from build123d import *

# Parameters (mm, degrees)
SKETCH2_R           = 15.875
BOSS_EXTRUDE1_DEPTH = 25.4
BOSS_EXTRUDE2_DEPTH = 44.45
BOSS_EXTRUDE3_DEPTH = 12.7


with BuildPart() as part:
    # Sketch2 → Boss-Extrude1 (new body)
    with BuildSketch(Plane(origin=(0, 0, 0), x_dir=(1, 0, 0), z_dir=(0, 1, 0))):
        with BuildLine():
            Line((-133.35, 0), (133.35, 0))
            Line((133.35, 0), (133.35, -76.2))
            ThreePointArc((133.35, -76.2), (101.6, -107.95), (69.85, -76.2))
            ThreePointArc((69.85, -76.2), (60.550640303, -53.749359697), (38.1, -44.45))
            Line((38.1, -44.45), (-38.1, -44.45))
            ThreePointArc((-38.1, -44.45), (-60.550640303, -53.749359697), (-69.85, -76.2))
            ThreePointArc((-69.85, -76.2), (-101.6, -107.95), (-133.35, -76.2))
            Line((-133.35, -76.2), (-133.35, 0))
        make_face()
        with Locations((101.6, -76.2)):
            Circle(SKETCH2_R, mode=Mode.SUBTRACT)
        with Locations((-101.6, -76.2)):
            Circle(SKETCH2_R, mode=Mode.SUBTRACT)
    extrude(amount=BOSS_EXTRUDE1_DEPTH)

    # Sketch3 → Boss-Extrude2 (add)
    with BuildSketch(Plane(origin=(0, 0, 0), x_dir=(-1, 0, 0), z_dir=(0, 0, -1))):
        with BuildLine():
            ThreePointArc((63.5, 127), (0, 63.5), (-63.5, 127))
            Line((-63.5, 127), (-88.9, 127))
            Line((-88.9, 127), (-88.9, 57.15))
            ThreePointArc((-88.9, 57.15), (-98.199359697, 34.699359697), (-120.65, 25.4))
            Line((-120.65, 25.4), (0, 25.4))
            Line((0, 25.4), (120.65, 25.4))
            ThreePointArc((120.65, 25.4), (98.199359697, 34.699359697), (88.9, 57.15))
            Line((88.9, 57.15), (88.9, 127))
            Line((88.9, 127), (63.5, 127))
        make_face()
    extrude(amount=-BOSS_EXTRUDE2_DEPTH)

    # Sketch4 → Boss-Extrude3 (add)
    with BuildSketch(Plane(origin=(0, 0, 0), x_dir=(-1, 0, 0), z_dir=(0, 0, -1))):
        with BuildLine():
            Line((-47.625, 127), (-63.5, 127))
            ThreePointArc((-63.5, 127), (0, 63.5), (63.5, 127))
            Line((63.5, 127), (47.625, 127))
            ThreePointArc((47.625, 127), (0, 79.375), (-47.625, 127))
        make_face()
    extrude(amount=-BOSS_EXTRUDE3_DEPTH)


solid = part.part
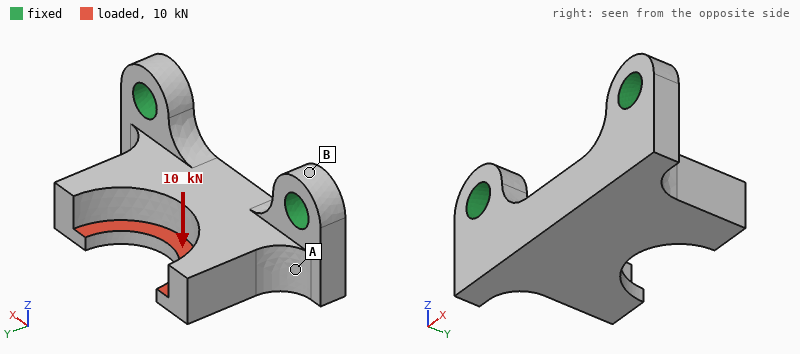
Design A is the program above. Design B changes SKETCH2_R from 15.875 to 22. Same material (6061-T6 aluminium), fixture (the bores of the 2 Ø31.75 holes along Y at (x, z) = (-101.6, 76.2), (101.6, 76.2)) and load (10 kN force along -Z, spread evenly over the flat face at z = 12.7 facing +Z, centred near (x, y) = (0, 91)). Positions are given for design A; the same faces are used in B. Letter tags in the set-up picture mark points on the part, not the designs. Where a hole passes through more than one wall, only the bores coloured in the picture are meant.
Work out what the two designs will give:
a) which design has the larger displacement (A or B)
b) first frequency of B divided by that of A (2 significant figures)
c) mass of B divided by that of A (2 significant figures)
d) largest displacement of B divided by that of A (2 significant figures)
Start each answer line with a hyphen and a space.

- A
- 1.1
- 0.96
- 0.83
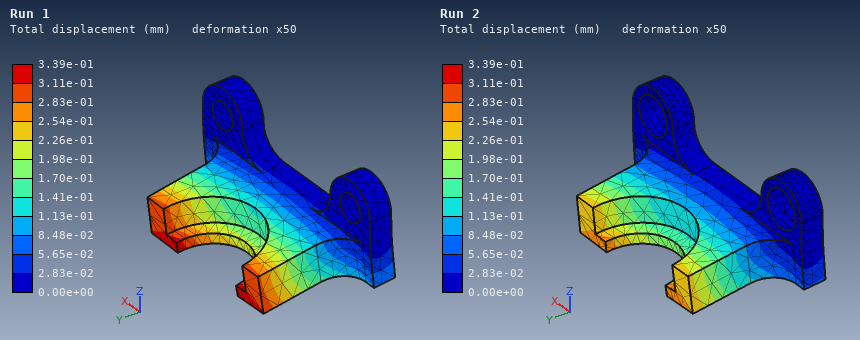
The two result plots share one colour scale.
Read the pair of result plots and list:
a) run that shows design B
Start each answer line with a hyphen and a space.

- Run 2
